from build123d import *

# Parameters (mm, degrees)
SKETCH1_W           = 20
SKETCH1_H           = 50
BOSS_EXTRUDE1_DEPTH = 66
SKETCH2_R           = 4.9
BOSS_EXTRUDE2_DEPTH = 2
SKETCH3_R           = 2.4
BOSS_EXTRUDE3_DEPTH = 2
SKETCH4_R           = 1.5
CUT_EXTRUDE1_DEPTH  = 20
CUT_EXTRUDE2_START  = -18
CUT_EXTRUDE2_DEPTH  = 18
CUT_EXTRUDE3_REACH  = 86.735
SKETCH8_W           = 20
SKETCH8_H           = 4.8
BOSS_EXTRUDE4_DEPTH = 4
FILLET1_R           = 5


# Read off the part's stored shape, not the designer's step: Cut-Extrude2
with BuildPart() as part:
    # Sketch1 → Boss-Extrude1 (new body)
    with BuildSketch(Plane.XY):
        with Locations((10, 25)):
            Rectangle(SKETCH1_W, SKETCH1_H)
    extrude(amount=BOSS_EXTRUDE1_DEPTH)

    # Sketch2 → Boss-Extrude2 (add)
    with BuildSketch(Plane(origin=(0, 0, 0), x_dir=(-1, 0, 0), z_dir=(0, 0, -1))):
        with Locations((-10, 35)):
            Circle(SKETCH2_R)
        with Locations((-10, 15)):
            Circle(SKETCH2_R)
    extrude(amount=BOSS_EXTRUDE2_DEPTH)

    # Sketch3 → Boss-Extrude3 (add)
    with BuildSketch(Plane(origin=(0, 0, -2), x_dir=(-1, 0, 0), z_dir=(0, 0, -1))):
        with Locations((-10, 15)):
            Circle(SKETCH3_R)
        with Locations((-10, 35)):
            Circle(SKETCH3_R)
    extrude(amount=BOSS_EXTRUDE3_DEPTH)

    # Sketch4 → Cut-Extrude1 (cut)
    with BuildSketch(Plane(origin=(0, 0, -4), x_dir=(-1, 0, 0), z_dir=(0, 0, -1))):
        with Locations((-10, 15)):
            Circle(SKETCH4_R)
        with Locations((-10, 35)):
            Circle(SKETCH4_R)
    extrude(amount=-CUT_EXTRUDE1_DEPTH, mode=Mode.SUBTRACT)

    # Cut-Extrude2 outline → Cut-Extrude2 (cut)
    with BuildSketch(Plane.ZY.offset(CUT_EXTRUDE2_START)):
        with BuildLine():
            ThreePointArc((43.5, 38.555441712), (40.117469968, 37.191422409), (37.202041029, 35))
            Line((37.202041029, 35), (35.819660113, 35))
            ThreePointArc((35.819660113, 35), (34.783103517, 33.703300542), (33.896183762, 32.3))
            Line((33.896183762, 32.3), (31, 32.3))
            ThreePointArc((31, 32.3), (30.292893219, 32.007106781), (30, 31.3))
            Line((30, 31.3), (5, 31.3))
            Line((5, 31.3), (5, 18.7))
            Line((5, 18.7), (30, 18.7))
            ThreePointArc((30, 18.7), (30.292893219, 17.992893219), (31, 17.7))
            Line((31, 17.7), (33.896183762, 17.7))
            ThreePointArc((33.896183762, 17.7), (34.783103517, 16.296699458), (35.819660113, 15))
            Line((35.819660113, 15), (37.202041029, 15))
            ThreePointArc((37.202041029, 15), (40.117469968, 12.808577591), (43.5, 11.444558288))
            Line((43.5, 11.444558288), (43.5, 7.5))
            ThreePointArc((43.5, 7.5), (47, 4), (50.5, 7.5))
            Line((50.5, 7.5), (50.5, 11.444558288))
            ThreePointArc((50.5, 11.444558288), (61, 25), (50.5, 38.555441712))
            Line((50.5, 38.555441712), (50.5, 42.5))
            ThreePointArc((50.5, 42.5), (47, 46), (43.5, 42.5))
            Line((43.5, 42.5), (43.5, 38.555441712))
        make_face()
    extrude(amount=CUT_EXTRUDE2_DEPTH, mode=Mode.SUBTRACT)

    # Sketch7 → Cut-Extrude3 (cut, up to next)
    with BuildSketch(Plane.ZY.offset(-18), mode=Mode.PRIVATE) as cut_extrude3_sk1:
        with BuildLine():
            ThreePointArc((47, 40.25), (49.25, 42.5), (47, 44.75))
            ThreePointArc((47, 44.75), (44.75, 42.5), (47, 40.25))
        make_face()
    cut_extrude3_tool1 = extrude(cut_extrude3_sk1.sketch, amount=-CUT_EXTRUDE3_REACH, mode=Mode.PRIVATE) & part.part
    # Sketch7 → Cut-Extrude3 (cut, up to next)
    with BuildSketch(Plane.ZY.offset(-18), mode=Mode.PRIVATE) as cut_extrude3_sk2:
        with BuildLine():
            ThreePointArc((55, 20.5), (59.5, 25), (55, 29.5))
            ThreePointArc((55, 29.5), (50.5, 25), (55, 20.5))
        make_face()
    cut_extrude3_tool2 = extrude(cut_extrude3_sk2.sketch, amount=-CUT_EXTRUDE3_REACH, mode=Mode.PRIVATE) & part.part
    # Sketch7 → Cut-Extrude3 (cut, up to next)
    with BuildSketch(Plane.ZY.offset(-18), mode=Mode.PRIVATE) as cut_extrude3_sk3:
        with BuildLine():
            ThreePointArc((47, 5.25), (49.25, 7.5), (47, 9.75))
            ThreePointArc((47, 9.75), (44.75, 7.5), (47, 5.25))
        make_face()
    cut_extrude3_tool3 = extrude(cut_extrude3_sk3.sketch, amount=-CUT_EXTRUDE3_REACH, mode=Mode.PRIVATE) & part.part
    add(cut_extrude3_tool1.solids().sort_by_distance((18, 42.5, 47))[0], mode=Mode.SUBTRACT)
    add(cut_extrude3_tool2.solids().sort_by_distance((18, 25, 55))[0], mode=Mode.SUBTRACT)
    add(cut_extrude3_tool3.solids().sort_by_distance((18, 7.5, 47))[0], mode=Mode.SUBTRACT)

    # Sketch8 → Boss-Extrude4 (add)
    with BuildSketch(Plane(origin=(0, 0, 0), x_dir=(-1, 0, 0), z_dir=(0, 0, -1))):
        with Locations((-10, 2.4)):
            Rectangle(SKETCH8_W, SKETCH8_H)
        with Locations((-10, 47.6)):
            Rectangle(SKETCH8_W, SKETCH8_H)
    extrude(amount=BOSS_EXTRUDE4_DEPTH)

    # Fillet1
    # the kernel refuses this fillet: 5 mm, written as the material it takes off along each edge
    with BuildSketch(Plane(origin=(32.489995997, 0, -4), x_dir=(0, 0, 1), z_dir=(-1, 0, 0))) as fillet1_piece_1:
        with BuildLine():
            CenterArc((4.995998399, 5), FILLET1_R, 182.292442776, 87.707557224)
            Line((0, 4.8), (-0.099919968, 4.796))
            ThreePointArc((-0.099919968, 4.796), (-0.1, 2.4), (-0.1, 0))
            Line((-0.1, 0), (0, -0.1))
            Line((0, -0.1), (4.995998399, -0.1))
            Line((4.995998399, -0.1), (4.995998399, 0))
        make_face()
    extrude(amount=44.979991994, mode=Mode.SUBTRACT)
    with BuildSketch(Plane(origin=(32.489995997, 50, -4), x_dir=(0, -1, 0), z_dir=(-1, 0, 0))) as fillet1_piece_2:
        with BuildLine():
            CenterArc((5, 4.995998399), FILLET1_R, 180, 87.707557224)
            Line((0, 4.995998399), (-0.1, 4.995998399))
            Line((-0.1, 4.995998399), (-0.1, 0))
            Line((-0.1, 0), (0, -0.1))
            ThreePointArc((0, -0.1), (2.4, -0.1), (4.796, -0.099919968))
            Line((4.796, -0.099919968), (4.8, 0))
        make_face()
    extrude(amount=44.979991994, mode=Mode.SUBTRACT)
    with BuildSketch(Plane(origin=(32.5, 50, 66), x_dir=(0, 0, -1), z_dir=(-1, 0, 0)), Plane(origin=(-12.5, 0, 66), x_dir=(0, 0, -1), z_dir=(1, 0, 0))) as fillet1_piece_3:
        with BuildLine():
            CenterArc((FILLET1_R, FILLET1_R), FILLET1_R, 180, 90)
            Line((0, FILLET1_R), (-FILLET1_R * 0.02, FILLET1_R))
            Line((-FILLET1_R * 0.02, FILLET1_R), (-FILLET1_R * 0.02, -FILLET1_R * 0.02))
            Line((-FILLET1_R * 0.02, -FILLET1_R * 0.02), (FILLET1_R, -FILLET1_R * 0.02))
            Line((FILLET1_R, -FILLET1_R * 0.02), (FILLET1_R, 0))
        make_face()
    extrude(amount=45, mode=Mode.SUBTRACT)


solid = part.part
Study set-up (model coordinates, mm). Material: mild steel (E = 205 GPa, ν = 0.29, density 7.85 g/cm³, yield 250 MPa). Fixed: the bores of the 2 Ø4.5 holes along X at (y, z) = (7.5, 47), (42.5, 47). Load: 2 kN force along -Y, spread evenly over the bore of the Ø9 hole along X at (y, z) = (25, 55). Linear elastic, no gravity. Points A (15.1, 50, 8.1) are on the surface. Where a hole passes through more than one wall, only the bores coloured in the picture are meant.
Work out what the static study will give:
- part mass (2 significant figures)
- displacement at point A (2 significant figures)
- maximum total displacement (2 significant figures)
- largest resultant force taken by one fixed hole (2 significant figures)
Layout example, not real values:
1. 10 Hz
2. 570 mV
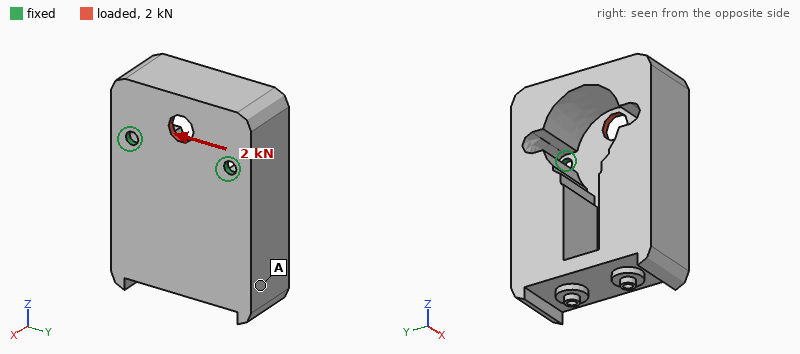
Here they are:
1. 370 g
2. 1.5 µm
3. 3.7 µm
4. 1.1 kN
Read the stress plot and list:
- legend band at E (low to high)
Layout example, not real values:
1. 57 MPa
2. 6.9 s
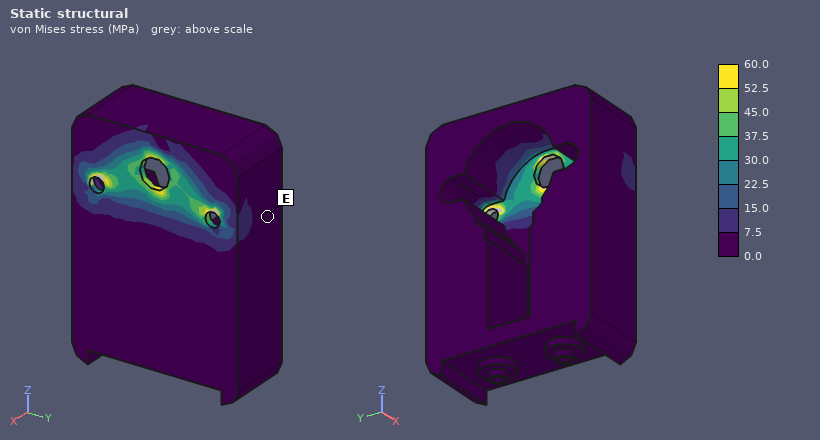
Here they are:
1. 0.0 to 7.5 MPa
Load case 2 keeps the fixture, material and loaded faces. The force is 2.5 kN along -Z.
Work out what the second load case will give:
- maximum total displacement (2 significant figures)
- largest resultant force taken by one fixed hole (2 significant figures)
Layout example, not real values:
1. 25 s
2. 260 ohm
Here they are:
1. 5.5 µm
2. 1.3 kN
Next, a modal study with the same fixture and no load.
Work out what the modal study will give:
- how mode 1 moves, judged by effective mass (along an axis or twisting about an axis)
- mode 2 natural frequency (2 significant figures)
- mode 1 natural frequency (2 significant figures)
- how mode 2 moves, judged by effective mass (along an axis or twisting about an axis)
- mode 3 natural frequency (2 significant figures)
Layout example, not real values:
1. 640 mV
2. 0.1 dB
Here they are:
1. along X
2. 3800 Hz
3. 860 Hz
4. along Y
5. 5600 Hz
